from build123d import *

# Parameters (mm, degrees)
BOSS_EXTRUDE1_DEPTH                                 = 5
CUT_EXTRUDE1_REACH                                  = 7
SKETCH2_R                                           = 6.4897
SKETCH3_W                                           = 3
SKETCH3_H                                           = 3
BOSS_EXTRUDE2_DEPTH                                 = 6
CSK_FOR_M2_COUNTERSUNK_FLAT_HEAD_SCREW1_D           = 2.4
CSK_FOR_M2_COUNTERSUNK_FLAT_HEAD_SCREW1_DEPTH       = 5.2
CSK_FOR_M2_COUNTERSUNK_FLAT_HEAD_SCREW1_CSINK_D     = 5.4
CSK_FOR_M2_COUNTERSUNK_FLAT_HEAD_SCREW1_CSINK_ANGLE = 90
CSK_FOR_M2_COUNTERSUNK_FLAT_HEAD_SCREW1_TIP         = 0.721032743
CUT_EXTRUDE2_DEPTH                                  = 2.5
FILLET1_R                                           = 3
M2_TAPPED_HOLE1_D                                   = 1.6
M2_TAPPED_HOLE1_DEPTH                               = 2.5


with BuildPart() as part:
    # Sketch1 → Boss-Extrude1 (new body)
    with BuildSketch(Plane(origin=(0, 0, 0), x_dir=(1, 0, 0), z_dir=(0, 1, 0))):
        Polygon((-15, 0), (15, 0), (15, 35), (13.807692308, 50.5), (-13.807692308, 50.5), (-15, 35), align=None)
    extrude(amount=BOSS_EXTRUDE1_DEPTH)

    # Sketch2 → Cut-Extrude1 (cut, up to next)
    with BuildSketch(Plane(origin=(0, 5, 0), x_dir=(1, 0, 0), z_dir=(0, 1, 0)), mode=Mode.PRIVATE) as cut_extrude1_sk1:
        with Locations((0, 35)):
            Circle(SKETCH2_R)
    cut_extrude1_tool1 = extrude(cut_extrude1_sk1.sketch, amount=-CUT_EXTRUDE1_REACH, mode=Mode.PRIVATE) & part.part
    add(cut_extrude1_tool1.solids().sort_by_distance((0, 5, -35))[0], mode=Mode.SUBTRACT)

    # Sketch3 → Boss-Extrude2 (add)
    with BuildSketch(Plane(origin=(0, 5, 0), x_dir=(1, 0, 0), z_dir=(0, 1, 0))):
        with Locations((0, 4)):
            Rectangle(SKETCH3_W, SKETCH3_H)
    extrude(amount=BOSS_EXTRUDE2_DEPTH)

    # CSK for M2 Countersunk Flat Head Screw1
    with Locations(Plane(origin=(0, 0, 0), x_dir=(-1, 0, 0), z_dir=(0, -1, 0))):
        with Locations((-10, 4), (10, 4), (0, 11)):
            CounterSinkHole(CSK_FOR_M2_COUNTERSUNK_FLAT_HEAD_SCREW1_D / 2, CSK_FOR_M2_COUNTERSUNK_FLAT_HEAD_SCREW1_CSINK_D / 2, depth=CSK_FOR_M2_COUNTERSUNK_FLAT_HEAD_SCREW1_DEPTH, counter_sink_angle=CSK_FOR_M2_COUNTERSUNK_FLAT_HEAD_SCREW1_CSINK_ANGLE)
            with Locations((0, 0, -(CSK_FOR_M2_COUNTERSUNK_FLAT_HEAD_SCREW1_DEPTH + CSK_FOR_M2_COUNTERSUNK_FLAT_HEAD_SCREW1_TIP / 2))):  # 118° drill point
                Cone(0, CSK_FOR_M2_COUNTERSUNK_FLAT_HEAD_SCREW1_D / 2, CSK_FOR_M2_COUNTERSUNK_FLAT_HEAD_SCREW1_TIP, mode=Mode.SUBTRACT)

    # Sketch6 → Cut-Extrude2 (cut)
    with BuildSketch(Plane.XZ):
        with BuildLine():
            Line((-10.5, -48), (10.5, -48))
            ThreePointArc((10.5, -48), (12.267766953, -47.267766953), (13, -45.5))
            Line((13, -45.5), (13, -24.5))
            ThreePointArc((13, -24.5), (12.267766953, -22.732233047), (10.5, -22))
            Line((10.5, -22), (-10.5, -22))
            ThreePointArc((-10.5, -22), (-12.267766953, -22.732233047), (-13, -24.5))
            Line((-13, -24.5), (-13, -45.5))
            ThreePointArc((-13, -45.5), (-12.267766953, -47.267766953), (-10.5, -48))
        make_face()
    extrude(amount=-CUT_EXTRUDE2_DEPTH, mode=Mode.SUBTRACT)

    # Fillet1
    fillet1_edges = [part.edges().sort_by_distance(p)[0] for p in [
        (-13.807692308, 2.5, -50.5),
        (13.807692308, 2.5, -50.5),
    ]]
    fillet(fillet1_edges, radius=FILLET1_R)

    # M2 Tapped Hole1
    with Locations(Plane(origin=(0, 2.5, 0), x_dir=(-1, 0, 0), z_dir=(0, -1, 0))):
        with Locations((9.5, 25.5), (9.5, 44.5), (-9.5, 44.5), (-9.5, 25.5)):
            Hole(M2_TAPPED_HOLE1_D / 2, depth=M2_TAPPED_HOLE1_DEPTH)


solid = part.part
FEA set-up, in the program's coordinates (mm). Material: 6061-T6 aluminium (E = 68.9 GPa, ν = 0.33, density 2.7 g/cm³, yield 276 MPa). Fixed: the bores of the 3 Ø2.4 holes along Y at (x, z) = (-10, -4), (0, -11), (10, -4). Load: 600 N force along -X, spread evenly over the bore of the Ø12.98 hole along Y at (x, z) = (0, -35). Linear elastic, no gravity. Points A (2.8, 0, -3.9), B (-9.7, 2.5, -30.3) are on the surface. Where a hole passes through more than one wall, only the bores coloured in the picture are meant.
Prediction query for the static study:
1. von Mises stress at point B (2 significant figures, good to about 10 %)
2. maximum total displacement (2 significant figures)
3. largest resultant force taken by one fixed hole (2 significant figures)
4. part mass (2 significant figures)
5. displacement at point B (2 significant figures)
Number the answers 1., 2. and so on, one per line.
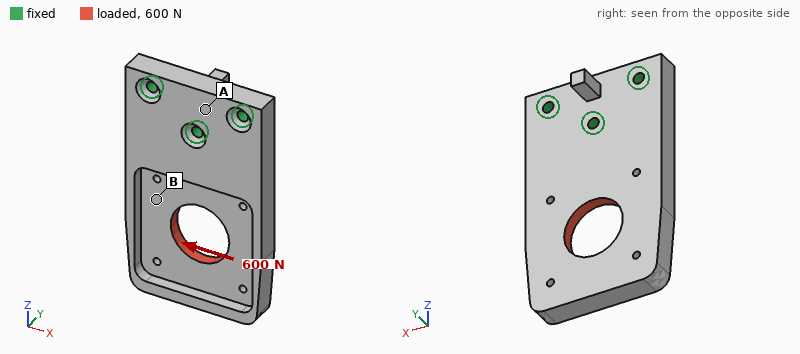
1. 20 MPa
2. 35 µm
3. 670 N
4. 15 g
5. 15 µm
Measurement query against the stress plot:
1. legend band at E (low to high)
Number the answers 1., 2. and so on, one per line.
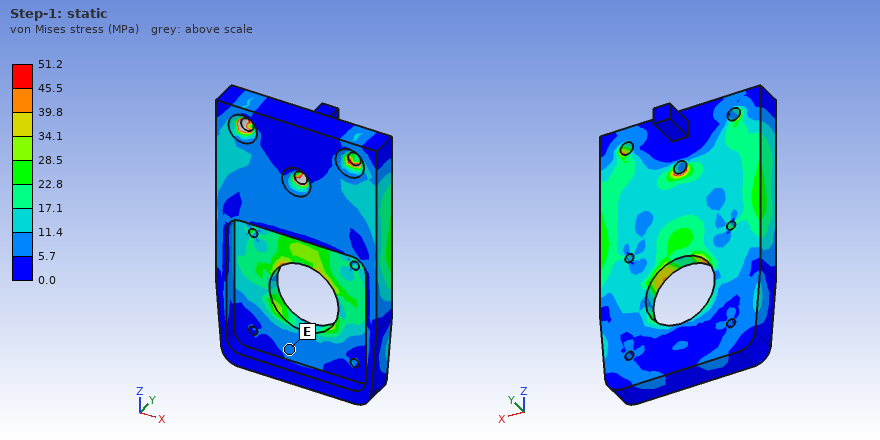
1. 5.7 to 11.4 MPa
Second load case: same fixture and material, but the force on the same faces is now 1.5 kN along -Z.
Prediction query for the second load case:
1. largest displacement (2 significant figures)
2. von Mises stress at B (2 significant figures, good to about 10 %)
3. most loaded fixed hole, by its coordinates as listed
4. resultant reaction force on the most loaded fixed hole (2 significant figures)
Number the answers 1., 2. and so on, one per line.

1. 56 µm
2. 22 MPa
3. (0, -11)
4. 650 N
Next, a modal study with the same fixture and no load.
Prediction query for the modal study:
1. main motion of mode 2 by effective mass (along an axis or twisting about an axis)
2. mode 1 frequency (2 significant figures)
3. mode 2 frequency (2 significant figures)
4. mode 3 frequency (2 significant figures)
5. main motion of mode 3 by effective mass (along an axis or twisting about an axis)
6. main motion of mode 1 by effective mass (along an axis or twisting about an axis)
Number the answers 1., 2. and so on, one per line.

1. twisting about Z
2. 2300 Hz
3. 4600 Hz
4. 9600 Hz
5. along X
6. along Y
